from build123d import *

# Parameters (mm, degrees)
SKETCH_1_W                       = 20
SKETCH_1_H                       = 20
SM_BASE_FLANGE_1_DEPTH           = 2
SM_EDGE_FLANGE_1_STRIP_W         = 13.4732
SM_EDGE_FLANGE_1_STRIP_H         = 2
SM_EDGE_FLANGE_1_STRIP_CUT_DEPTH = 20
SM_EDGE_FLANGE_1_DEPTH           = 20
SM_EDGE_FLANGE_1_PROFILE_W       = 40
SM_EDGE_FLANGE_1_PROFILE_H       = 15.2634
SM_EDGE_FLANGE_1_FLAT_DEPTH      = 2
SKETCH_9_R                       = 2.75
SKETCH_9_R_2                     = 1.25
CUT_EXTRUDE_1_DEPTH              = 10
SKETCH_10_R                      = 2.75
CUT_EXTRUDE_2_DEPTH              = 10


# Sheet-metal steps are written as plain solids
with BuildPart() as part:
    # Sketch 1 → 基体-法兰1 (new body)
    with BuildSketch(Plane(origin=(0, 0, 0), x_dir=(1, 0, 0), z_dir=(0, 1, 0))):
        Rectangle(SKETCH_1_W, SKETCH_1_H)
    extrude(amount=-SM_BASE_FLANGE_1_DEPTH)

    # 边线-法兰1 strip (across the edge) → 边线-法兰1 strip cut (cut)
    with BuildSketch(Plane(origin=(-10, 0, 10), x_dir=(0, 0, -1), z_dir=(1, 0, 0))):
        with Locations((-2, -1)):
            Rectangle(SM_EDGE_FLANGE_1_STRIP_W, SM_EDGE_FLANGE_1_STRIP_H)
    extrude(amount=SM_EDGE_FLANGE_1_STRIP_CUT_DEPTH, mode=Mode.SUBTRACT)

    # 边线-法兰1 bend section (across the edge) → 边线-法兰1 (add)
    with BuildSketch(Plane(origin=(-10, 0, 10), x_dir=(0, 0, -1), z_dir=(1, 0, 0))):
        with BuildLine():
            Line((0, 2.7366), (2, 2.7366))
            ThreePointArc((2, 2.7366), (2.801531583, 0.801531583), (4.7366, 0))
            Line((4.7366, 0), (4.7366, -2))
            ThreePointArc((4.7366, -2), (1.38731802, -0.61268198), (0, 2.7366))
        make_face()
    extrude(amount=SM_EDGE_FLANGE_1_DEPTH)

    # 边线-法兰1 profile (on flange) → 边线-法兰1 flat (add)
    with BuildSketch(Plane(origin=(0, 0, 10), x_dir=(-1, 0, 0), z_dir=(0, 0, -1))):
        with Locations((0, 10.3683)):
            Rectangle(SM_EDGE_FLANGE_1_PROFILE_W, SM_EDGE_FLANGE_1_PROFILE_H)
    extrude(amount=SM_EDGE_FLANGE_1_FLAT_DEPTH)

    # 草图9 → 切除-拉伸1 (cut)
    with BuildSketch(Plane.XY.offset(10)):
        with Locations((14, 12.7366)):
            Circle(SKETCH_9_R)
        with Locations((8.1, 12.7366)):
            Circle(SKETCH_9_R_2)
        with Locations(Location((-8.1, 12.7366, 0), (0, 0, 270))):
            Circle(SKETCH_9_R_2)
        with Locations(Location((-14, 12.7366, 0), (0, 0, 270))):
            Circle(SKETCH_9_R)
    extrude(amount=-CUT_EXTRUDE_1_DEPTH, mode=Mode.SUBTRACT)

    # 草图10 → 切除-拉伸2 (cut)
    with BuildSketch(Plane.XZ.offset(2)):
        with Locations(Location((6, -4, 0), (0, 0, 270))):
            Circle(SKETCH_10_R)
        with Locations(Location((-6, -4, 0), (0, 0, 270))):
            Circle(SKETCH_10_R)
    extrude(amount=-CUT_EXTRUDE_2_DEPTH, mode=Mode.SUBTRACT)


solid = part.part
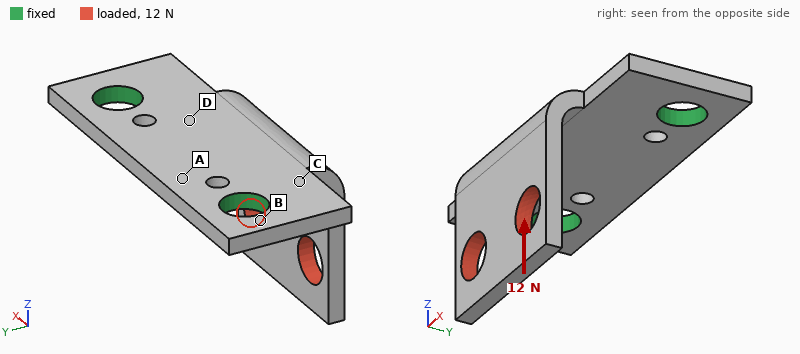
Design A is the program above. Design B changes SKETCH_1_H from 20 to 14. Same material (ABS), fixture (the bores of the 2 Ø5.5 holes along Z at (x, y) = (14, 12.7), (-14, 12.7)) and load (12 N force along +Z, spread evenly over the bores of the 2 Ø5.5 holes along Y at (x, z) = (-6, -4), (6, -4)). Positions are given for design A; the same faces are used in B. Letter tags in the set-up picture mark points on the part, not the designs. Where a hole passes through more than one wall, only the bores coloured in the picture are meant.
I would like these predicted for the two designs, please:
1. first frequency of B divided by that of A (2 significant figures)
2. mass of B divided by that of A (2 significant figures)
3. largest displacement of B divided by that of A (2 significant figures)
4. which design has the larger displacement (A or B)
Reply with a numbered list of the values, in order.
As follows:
1. 1.3
2. 0.94
3. 0.89
4. A
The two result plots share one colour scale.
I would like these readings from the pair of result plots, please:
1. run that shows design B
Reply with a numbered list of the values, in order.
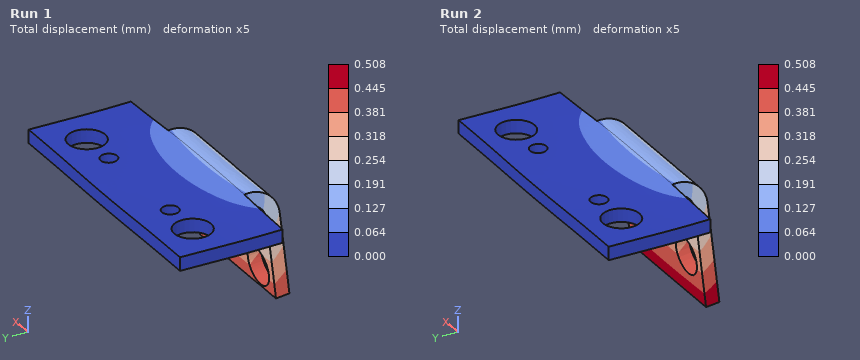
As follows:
1. Run 1
